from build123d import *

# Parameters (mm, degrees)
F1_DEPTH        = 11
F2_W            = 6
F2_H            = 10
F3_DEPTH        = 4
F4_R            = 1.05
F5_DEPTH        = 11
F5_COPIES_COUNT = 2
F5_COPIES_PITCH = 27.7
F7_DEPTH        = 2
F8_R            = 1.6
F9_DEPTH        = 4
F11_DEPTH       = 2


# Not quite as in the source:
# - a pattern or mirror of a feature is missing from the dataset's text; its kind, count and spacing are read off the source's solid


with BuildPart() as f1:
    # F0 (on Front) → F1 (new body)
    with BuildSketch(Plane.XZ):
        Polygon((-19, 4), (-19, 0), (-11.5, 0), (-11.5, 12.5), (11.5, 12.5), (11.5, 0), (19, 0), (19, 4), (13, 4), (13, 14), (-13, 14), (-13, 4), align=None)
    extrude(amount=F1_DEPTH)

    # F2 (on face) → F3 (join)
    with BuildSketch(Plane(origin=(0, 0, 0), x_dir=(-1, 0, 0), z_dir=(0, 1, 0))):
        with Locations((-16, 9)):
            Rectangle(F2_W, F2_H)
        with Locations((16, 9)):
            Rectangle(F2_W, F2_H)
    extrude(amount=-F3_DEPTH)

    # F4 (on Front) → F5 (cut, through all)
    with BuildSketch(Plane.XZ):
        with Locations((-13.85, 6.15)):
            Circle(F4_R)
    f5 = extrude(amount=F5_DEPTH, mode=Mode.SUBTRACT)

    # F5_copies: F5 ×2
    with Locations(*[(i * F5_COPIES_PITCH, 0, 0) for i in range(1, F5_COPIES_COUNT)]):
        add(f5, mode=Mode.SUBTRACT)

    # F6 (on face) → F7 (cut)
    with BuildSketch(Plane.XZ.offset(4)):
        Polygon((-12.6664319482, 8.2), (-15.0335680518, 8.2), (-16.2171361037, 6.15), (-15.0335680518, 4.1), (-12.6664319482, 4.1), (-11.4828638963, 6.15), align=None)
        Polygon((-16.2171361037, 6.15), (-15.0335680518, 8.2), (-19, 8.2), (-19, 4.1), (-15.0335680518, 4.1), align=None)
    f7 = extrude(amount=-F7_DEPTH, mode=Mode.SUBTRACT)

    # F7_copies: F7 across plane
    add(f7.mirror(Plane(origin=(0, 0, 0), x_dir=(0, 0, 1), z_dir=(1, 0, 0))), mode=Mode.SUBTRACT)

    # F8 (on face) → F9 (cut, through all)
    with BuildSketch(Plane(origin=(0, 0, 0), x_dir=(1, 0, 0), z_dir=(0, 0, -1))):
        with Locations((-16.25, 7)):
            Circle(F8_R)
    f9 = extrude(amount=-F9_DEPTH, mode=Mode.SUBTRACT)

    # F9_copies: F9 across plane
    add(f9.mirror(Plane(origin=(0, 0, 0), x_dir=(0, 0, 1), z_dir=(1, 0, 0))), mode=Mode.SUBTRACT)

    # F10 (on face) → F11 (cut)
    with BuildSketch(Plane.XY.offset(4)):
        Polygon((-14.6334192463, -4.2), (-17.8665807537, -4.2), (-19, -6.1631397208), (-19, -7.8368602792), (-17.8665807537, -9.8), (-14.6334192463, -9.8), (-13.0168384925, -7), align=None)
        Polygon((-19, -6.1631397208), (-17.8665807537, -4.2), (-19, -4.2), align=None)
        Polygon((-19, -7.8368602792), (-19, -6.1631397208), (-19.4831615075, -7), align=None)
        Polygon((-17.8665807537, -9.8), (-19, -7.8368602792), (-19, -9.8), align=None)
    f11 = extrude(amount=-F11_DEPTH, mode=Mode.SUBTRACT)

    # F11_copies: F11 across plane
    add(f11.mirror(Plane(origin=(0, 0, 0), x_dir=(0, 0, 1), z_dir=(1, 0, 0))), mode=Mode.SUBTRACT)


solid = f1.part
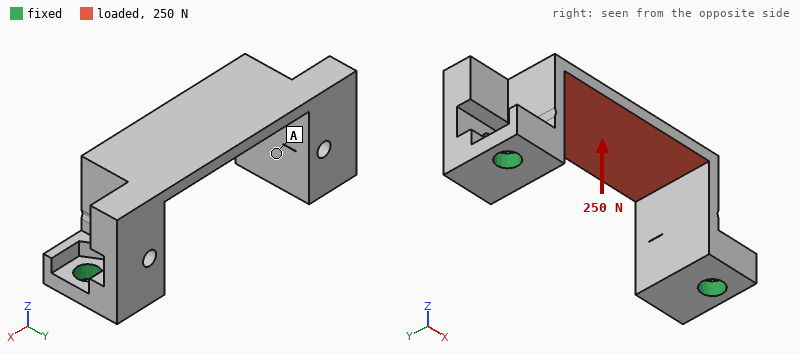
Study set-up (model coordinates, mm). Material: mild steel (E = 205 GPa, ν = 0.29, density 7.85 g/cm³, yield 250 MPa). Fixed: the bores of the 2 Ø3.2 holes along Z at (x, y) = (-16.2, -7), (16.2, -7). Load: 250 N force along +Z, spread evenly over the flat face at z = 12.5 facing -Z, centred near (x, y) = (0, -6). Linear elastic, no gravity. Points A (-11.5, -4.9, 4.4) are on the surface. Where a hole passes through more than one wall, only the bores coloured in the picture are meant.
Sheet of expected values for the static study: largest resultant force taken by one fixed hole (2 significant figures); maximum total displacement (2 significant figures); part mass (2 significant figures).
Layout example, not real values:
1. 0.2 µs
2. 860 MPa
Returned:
1. 140 N
2. 22 µm
3. 12 g
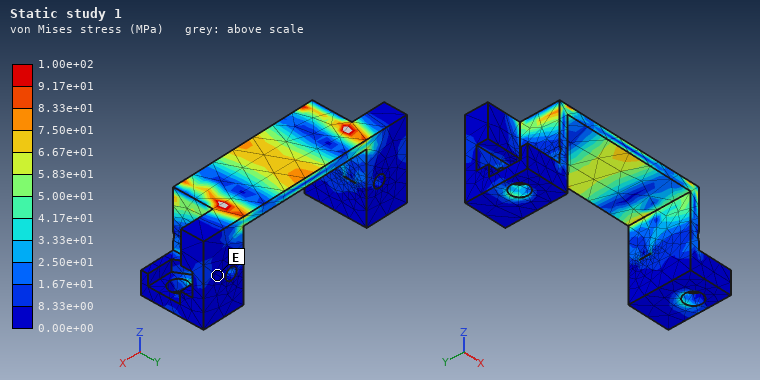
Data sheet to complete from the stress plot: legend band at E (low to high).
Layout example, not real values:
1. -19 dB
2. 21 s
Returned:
1. 0.00e+00 to 8.33e+00 MPa
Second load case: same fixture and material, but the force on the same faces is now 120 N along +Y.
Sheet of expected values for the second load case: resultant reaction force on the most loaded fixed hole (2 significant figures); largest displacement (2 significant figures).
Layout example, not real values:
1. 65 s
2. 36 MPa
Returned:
1. 62 N
2. 8.4 µm
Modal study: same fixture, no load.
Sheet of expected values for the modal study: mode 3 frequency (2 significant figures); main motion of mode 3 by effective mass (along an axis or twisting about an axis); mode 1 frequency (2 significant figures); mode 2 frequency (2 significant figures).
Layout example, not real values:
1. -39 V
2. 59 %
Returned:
1. 9300 Hz
2. twisting about Z
3. 7600 Hz
4. 7600 Hz
